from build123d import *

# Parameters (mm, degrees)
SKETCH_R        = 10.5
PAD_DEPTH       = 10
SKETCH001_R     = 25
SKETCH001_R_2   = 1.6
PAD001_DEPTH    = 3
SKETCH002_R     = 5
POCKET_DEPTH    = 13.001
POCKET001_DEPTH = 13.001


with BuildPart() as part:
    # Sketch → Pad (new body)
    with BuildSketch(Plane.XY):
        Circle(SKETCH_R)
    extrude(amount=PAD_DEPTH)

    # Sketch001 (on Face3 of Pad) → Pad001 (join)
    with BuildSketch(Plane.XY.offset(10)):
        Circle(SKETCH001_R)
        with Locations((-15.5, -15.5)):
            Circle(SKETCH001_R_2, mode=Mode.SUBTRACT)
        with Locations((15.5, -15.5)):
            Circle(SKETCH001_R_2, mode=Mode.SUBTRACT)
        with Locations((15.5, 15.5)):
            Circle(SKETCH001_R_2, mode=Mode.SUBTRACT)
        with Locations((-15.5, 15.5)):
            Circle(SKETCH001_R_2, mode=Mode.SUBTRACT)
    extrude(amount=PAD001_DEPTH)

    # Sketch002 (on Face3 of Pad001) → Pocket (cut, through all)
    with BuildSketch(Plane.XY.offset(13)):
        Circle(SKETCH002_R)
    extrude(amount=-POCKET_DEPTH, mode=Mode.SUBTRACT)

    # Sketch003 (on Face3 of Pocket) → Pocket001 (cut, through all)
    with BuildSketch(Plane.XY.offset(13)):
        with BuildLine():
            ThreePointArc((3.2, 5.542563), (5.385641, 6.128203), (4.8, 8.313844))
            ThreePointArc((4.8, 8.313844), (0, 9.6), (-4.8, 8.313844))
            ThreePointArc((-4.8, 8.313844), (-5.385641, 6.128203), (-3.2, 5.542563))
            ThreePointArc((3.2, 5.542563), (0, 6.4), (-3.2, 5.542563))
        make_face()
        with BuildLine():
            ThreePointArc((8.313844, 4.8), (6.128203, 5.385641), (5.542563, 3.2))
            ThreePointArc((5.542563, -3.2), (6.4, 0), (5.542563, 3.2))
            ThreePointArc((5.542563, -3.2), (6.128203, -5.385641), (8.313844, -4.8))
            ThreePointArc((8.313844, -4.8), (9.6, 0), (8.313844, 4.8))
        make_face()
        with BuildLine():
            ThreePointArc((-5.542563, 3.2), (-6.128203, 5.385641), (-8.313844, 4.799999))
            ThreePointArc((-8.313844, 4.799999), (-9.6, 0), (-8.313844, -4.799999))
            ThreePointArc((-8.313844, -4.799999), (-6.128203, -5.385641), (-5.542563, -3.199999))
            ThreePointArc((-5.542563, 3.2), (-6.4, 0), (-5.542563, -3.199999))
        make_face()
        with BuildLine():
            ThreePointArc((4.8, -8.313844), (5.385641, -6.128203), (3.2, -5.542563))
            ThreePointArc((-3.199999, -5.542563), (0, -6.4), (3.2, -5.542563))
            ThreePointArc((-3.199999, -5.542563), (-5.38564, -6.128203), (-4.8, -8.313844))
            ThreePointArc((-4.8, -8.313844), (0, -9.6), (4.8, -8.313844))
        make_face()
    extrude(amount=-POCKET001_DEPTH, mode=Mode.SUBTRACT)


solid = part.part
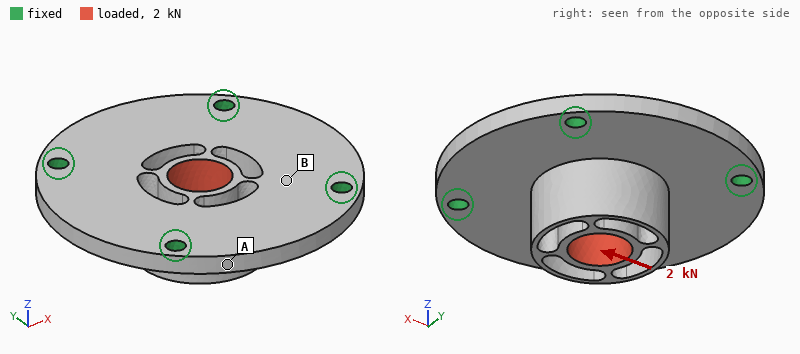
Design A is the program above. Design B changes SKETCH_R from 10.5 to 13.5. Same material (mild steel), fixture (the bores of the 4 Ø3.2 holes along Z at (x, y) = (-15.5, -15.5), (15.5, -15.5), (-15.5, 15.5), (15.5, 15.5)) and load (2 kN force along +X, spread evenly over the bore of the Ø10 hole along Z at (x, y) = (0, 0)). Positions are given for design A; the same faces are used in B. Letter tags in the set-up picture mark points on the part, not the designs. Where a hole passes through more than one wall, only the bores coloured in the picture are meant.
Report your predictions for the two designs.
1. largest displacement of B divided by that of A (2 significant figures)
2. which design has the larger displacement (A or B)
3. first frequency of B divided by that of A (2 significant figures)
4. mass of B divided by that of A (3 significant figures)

0.54
A
1.0
1.35
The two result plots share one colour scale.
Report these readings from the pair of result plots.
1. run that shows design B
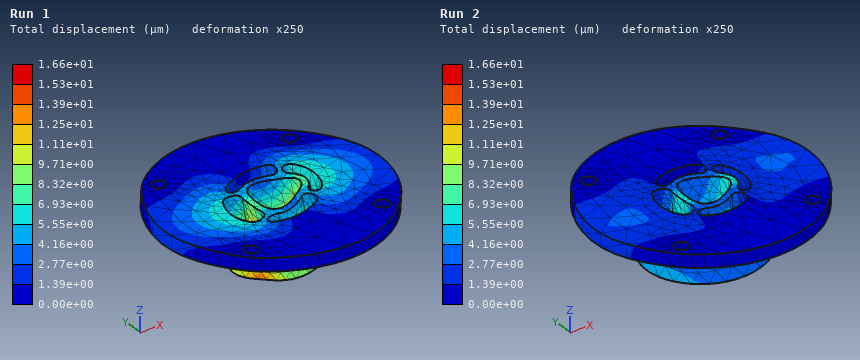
Run 2
